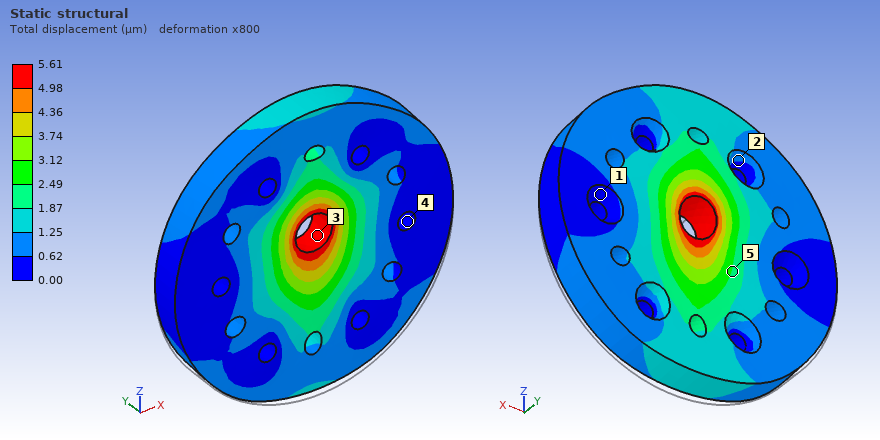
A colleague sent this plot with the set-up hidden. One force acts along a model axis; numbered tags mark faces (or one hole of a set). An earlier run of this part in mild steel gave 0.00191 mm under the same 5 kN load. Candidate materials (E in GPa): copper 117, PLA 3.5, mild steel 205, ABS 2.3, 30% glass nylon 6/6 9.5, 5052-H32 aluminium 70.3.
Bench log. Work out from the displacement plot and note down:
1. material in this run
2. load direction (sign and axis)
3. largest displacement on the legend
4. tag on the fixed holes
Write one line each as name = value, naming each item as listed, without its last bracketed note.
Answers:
material in this run = 5052-H32 aluminium
load direction = +Z
largest displacement on the legend = 5.61 µm
tag on the fixed holes = 4
